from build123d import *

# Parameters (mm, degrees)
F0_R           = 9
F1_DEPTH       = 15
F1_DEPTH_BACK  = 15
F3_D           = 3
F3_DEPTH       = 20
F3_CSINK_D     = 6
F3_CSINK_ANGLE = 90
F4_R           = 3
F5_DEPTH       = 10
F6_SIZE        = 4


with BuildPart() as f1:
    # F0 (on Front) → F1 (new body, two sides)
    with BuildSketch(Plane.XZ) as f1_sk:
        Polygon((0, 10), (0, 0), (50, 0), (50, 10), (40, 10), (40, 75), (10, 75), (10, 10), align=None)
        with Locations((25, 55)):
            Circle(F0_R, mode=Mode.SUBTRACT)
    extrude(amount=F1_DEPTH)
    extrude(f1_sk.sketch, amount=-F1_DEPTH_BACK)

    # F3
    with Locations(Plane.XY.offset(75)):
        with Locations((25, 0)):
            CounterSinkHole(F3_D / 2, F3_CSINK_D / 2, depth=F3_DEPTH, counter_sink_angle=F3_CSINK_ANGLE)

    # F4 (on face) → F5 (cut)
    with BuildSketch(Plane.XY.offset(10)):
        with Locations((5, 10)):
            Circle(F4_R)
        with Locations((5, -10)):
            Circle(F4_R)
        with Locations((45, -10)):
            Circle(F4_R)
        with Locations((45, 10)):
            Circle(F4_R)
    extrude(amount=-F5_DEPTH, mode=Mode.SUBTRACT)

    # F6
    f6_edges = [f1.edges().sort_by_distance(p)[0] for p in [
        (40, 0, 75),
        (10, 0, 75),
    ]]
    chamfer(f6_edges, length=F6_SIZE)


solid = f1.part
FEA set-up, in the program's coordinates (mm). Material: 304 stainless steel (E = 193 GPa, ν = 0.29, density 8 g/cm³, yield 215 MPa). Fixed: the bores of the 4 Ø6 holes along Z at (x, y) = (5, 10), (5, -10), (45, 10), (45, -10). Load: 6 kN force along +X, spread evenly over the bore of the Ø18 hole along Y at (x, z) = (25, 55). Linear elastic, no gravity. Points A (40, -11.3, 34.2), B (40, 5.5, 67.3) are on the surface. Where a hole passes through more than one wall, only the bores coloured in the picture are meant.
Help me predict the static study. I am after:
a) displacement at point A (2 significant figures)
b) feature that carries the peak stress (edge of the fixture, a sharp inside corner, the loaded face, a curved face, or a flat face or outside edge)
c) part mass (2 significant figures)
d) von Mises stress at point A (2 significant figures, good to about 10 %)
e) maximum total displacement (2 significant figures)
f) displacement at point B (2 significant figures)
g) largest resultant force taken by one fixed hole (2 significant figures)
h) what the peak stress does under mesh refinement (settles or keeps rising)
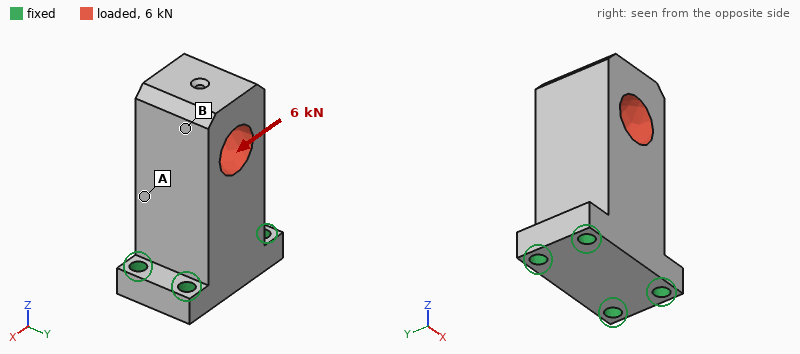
17 µm
edge of the fixture
510 g
30 MPa
51 µm
46 µm
4.7 kN
keeps rising
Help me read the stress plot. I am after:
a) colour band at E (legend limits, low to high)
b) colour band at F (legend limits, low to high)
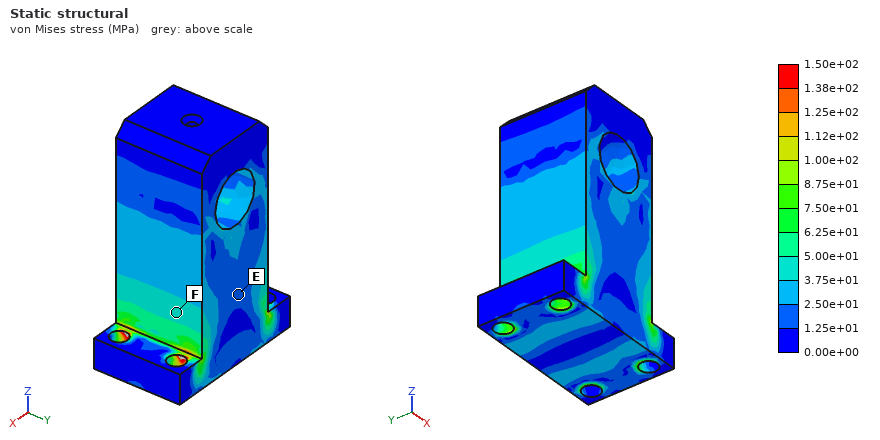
1.25e+01 to 2.50e+01 MPa
3.75e+01 to 5.00e+01 MPa
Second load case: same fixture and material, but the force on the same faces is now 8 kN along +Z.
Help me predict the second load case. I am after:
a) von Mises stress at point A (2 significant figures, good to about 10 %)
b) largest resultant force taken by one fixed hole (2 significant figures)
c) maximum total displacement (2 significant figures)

11 MPa
2.1 kN
5.6 µm
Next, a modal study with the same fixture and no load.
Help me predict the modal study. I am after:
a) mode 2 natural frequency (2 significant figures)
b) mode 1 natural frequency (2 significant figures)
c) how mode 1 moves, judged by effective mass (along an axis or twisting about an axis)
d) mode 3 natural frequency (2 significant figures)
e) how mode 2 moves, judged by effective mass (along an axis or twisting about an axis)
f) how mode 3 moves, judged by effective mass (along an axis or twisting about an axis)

4100 Hz
3200 Hz
along Y
10000 Hz
along X
twisting about Z
